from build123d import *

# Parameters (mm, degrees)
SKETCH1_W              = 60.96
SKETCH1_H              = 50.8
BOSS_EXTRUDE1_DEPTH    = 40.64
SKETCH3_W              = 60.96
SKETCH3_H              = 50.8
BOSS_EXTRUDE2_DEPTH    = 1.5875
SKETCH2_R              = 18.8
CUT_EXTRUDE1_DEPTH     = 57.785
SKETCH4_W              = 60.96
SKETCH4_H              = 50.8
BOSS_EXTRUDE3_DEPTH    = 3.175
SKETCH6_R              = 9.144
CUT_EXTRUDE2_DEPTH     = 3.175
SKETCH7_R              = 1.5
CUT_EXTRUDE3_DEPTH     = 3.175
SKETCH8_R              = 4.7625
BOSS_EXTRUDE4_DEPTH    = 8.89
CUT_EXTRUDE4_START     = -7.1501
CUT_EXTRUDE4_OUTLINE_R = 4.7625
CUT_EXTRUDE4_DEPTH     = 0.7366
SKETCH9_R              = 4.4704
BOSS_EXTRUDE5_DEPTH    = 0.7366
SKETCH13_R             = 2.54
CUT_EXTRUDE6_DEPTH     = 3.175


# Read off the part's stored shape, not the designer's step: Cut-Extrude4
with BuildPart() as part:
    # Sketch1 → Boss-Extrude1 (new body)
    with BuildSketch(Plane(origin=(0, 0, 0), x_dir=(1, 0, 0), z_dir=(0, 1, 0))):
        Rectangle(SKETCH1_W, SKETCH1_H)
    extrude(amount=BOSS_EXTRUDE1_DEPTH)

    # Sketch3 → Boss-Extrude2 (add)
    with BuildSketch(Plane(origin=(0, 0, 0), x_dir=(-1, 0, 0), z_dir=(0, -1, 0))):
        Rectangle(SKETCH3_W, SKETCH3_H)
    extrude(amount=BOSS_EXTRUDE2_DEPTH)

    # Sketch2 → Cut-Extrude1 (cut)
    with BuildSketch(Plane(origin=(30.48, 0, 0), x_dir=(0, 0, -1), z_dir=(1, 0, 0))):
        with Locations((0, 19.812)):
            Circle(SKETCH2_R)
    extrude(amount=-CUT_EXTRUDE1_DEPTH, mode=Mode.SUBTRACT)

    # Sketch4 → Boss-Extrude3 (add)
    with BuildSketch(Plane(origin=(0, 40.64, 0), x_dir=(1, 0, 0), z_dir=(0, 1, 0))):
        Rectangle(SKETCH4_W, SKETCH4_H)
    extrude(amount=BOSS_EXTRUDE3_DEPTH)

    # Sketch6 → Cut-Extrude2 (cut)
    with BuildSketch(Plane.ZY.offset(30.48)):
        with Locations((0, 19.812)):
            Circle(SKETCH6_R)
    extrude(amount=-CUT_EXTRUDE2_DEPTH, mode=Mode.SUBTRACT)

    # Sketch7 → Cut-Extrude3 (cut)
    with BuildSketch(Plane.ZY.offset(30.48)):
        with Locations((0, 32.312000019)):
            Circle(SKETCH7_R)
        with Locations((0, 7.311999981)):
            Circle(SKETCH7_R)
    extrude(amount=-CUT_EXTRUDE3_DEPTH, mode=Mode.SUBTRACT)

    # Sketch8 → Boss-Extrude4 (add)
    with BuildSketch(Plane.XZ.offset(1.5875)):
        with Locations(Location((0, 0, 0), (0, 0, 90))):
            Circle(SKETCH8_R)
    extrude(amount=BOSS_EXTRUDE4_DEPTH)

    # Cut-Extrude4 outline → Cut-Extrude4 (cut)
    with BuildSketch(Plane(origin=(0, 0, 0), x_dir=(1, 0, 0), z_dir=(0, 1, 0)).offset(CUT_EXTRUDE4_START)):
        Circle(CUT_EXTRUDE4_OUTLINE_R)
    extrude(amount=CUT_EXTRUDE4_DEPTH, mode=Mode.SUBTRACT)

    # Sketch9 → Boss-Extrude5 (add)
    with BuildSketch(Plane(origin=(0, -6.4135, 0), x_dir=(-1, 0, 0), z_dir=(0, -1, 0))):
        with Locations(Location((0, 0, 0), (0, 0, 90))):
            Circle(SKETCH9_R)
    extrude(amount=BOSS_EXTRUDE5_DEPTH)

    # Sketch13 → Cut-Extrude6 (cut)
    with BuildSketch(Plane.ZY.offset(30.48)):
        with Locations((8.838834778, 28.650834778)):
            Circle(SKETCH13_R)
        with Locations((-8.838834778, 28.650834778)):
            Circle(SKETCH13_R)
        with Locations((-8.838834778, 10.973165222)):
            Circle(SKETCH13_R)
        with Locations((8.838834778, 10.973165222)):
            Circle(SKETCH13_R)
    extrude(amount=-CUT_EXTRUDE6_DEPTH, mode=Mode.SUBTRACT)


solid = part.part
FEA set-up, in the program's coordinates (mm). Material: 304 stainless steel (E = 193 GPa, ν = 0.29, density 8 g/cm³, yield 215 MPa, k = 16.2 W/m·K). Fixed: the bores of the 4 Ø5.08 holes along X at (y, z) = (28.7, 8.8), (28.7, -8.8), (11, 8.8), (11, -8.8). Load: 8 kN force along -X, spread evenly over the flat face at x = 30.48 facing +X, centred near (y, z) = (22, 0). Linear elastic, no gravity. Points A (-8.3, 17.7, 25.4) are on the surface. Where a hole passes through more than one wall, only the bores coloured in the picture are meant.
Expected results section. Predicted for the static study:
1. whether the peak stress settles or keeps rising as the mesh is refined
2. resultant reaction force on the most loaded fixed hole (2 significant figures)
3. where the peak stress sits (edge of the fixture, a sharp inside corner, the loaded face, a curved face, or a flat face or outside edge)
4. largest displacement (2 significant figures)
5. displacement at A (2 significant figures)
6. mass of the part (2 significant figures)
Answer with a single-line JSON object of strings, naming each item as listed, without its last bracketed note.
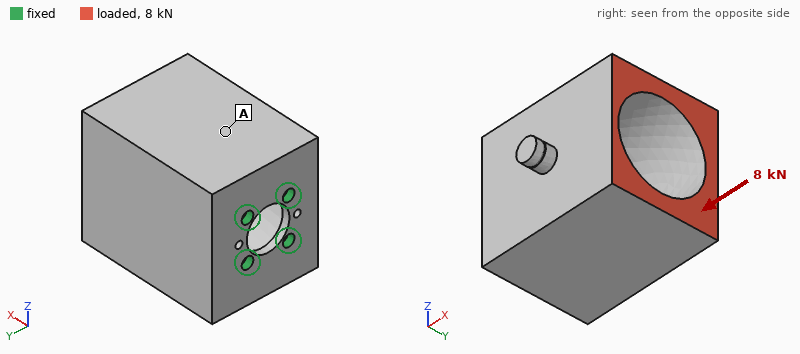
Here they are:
{"whether the peak stress settles or keeps rising as the mesh is refined": "keeps rising", "resultant reaction force on the most loaded fixed hole": "2.5 kN", "where the peak stress sits": "edge of the fixture", "largest displacement": "18 µm", "displacement at A": "10 µm", "mass of the part": "610 g"}
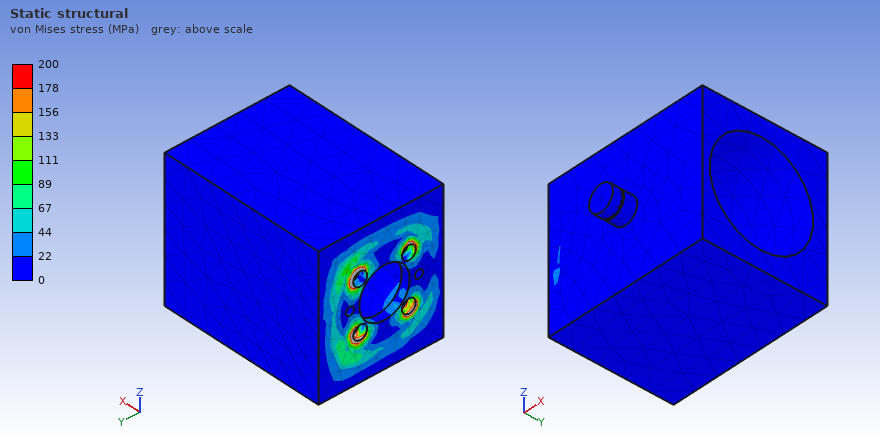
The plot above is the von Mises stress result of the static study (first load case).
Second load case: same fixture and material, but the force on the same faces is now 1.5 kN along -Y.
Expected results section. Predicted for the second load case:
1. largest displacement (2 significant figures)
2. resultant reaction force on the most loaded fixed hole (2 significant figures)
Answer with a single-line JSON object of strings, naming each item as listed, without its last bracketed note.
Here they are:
{"largest displacement": "55 µm", "resultant reaction force on the most loaded fixed hole": "1.9 kN"}
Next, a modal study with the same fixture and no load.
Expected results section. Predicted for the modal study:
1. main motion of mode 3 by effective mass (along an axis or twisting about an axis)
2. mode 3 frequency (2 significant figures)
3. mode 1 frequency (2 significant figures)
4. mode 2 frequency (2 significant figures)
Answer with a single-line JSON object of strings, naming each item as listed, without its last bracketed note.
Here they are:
{"main motion of mode 3 by effective mass": "along X", "mode 3 frequency": "5900 Hz", "mode 1 frequency": "1700 Hz", "mode 2 frequency": "1800 Hz"}
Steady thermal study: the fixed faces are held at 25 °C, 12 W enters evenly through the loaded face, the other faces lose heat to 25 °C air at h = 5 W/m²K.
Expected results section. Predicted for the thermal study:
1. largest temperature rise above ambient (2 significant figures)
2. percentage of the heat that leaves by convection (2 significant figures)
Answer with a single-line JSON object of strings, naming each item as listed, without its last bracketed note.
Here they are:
{"largest temperature rise above ambient": "47 K", "percentage of the heat that leaves by convection": "25 %"}
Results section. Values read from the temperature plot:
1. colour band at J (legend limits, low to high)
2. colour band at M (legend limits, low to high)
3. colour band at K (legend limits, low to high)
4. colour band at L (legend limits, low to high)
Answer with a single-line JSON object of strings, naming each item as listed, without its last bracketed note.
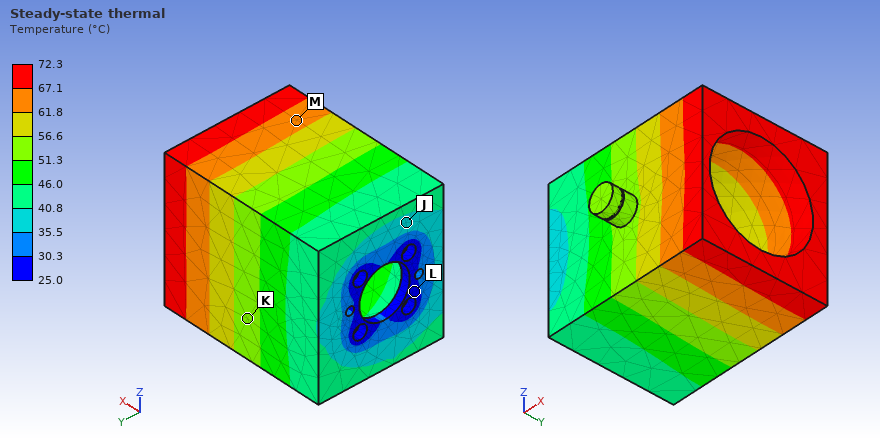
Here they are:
{"colour band at J": "35.5 to 40.8 °C", "colour band at M": "61.8 to 67.1 °C", "colour band at K": "51.3 to 56.6 °C", "colour band at L": "25.0 to 30.3 °C"}
